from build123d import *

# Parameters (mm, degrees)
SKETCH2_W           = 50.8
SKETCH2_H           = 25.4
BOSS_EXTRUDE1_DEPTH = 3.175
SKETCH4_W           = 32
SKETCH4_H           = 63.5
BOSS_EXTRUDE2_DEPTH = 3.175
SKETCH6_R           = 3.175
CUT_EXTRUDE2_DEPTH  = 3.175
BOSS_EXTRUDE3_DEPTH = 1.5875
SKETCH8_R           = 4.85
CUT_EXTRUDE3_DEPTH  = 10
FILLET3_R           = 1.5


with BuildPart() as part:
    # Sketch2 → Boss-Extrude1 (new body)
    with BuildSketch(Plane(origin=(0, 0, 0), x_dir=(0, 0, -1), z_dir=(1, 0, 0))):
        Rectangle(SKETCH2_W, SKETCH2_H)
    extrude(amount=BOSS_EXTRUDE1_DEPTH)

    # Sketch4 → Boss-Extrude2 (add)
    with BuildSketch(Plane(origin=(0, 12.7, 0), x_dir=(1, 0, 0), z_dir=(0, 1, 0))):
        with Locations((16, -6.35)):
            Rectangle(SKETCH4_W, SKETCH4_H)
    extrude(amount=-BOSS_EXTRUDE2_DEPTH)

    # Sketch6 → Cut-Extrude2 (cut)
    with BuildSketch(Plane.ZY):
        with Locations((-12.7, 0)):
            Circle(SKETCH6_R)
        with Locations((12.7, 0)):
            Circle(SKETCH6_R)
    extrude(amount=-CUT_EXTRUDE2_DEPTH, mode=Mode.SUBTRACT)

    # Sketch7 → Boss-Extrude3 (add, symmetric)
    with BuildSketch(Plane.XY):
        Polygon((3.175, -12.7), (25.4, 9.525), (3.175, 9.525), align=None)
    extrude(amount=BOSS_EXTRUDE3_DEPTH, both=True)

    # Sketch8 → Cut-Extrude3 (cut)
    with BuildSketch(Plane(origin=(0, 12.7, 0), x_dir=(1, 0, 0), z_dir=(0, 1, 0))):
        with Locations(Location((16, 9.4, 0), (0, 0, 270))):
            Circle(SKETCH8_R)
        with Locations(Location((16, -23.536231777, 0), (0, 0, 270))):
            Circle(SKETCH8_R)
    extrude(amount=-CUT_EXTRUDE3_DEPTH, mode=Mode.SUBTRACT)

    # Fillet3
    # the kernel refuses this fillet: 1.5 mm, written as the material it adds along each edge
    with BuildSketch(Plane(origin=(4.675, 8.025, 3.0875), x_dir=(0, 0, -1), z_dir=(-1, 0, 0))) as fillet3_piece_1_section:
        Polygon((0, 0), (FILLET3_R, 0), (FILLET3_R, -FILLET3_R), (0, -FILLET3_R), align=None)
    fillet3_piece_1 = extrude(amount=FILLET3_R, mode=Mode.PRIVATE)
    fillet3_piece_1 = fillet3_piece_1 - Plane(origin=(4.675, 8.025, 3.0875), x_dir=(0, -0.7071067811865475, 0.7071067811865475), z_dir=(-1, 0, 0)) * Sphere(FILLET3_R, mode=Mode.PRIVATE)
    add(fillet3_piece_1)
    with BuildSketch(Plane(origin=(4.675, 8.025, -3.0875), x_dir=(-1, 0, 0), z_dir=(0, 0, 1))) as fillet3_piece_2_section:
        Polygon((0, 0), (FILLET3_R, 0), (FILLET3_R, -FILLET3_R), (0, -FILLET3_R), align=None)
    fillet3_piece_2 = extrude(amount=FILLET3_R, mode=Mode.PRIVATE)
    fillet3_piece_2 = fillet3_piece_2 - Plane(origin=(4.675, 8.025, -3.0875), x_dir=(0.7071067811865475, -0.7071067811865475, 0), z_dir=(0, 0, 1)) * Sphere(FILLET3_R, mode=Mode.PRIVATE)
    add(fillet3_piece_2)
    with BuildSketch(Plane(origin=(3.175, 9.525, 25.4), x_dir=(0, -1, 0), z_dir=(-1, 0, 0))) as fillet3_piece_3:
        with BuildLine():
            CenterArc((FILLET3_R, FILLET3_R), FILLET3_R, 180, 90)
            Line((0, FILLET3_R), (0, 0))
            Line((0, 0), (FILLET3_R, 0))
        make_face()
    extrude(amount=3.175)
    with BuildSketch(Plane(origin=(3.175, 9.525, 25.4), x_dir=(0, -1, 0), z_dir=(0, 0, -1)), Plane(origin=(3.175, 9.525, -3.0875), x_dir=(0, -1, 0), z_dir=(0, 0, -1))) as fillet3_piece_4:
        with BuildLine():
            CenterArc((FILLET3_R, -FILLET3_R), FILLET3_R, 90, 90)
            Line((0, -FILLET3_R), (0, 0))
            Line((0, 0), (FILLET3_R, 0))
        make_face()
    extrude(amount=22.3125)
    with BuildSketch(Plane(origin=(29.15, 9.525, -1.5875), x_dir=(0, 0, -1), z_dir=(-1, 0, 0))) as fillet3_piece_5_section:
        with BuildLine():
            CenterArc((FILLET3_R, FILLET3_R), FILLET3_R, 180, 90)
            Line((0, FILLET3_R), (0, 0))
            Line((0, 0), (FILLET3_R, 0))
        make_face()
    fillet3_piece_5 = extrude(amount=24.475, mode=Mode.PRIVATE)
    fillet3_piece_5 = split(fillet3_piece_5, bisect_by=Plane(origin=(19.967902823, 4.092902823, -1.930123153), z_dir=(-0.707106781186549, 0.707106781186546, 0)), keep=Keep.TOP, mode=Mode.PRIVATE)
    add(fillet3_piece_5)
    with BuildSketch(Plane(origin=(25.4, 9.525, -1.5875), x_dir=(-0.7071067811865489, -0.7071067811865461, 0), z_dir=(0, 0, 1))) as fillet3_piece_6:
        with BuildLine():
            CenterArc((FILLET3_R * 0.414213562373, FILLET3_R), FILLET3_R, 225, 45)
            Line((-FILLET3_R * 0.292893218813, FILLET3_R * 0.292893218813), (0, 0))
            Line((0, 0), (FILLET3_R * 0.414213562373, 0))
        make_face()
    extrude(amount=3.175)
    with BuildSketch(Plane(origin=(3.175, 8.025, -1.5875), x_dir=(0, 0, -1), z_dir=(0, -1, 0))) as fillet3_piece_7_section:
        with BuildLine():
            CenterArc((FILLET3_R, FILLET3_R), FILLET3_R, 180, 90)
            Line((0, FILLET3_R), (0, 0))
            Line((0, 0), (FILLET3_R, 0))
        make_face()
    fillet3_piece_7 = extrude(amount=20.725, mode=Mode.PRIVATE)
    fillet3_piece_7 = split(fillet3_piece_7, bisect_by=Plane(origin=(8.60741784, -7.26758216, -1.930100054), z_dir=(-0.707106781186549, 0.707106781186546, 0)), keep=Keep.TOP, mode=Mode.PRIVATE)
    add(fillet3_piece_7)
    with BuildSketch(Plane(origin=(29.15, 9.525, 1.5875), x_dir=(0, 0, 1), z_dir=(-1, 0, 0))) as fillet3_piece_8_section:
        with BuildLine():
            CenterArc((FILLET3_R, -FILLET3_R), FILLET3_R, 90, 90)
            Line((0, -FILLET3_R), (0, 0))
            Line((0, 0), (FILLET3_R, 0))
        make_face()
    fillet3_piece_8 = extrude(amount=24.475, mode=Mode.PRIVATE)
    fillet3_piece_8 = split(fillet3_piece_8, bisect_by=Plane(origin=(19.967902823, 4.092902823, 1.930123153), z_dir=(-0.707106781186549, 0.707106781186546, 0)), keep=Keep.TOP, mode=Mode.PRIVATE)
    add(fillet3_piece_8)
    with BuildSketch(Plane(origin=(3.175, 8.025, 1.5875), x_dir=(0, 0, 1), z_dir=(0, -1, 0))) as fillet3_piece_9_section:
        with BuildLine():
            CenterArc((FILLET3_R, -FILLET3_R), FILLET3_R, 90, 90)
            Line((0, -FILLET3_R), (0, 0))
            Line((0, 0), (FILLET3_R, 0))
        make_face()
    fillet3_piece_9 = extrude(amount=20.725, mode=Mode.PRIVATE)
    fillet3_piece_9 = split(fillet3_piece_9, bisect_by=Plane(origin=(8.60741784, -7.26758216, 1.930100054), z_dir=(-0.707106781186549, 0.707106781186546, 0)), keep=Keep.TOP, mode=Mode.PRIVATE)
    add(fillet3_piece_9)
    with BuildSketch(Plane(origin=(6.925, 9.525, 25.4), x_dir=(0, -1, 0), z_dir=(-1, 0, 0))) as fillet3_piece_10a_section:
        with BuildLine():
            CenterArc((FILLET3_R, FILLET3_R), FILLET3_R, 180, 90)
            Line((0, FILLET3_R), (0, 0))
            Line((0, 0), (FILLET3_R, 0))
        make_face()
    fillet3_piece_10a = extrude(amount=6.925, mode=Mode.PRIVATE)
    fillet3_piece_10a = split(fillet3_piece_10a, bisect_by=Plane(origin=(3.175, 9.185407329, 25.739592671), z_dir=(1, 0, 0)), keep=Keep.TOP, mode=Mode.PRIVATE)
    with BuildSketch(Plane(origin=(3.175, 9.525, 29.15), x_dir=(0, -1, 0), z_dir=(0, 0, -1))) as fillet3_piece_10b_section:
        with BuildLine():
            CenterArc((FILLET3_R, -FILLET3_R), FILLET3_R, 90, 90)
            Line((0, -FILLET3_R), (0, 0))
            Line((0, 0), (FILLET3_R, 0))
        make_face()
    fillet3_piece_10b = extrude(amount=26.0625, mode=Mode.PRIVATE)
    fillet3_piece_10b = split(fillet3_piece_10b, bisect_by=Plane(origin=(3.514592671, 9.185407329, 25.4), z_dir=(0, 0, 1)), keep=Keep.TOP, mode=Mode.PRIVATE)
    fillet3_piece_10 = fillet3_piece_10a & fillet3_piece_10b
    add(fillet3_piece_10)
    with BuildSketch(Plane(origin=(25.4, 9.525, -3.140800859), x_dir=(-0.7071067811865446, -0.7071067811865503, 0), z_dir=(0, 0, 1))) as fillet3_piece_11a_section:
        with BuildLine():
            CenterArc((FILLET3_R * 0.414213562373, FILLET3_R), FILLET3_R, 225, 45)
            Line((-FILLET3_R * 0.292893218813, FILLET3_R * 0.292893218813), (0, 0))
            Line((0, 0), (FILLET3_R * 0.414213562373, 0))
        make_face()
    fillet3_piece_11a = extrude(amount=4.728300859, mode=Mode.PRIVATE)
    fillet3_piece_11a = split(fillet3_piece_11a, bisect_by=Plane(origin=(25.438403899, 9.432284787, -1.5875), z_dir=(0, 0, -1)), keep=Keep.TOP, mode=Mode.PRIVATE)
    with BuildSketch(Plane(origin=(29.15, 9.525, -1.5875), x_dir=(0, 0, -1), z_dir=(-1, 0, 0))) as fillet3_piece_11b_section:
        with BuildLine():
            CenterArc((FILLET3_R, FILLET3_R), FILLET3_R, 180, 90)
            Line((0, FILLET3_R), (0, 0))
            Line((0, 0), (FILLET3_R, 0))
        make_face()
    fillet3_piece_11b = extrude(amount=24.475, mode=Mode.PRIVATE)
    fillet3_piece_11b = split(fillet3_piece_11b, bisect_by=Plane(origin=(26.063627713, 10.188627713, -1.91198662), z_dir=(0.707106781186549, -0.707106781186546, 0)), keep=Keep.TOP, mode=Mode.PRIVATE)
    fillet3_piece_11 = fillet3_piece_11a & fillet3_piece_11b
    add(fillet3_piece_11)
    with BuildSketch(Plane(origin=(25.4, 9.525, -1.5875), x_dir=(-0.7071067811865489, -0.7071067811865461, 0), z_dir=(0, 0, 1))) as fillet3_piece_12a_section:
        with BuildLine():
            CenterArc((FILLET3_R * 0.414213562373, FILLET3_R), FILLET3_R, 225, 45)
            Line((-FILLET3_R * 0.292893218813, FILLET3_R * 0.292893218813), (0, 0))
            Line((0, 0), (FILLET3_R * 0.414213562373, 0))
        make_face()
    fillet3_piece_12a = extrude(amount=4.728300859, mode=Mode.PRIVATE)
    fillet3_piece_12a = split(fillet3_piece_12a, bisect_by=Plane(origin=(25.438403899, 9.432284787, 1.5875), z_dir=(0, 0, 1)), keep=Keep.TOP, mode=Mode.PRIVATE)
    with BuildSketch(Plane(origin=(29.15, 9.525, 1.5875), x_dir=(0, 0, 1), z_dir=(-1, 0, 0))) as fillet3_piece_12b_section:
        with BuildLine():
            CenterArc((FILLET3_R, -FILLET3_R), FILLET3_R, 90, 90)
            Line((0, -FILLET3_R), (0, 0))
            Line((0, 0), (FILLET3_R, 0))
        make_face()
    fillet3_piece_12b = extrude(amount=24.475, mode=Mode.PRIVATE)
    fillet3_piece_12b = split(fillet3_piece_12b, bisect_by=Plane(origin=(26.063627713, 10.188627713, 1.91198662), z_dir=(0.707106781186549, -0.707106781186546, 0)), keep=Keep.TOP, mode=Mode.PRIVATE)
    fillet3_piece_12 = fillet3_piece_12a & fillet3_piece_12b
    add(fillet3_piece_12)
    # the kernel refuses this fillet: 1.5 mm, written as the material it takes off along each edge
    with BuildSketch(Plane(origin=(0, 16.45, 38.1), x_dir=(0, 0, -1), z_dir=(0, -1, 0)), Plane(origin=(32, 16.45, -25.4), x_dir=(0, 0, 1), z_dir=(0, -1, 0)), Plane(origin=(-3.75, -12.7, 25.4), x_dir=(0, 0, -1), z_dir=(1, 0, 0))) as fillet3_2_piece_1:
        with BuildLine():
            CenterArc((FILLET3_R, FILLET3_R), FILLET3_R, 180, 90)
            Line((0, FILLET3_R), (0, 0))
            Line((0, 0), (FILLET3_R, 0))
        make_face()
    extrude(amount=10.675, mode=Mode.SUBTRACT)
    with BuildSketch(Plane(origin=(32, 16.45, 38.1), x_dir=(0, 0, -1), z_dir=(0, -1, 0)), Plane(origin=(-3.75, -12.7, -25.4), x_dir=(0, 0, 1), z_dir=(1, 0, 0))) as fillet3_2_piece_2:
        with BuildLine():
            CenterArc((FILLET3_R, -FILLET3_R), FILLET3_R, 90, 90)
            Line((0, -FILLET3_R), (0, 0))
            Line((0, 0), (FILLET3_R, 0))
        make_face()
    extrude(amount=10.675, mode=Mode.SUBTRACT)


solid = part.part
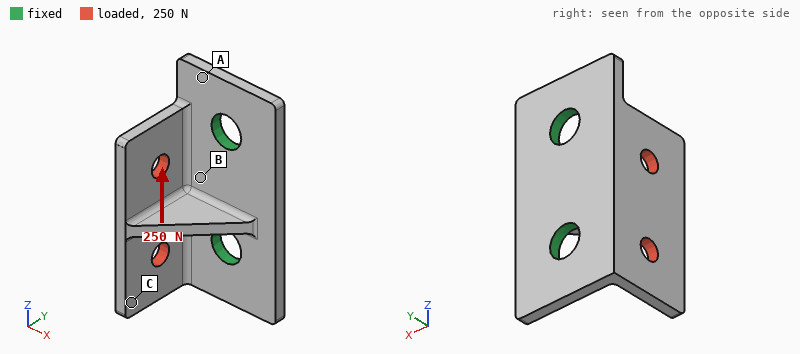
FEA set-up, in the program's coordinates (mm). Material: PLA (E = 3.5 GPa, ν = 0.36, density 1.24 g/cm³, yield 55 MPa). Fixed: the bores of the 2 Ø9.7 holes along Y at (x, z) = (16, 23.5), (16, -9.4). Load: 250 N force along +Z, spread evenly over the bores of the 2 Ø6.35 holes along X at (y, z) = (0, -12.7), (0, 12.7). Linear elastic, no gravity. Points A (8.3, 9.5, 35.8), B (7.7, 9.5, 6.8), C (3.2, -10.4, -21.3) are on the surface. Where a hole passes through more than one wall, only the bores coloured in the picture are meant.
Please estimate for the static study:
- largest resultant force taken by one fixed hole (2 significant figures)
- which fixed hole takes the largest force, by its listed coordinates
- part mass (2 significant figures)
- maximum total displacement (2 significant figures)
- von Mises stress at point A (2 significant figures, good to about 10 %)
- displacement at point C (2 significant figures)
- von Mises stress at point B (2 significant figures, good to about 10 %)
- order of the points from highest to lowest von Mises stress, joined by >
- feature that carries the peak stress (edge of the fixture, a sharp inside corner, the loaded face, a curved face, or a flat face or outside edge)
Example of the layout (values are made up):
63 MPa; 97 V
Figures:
180 N; (16, -9.4); 13 g; 0.23 mm; 3.4 MPa; 0.21 mm; 5.4 MPa; B > A > C; a curved face
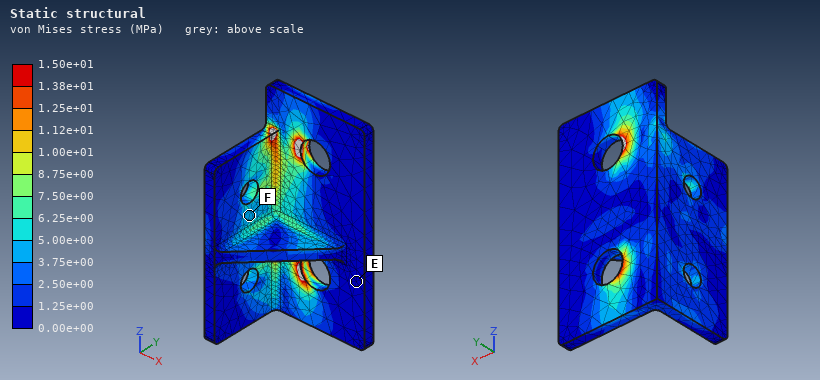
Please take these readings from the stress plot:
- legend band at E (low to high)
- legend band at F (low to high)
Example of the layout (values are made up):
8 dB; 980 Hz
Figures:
0.00e+00 to 1.25e+00 MPa; 3.75e+00 to 5.00e+00 MPa
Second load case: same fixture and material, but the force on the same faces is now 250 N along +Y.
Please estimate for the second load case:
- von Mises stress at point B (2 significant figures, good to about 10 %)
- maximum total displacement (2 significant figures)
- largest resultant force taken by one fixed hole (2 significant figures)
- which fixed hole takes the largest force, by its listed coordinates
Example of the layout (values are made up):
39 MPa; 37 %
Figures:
2.0 MPa; 0.42 mm; 180 N; (16, -9.4)
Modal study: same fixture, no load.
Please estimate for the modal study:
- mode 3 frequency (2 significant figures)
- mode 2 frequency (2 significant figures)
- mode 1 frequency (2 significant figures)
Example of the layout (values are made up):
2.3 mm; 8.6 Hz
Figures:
2800 Hz; 1900 Hz; 1600 Hz
